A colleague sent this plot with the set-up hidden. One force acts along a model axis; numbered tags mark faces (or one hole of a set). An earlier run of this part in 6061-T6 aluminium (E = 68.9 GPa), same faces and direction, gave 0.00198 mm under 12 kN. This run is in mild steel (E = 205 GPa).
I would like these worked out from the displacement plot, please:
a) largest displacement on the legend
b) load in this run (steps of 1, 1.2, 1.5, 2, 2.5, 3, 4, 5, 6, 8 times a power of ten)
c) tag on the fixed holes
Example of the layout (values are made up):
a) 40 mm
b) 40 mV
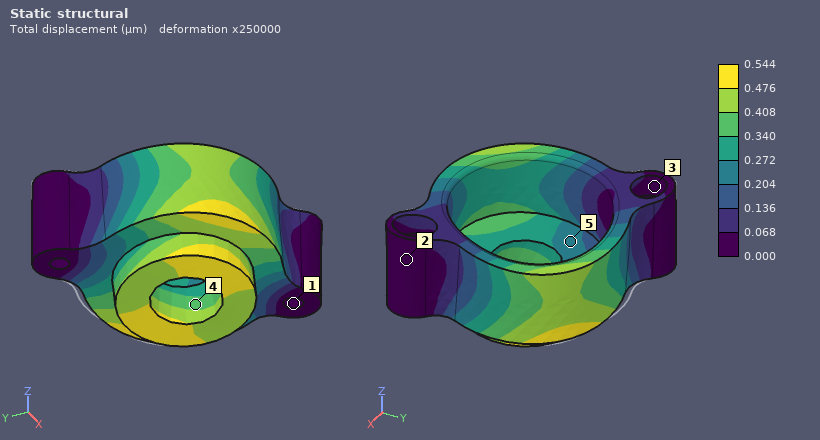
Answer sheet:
a) 0.544 µm
b) 10 kN
c) 1
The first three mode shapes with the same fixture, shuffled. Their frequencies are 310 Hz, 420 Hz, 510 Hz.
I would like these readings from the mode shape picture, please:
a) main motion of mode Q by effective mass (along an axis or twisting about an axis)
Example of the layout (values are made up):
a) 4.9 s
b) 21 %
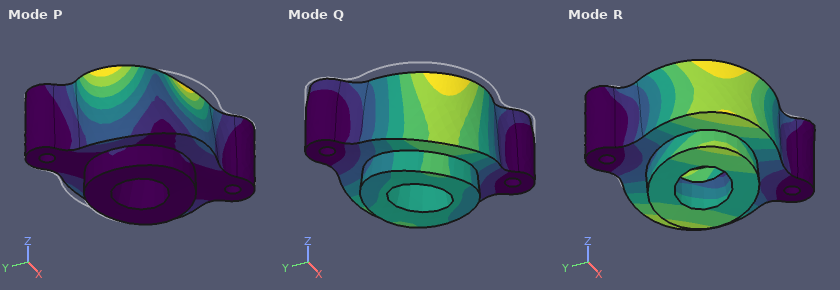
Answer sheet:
a) along Z
